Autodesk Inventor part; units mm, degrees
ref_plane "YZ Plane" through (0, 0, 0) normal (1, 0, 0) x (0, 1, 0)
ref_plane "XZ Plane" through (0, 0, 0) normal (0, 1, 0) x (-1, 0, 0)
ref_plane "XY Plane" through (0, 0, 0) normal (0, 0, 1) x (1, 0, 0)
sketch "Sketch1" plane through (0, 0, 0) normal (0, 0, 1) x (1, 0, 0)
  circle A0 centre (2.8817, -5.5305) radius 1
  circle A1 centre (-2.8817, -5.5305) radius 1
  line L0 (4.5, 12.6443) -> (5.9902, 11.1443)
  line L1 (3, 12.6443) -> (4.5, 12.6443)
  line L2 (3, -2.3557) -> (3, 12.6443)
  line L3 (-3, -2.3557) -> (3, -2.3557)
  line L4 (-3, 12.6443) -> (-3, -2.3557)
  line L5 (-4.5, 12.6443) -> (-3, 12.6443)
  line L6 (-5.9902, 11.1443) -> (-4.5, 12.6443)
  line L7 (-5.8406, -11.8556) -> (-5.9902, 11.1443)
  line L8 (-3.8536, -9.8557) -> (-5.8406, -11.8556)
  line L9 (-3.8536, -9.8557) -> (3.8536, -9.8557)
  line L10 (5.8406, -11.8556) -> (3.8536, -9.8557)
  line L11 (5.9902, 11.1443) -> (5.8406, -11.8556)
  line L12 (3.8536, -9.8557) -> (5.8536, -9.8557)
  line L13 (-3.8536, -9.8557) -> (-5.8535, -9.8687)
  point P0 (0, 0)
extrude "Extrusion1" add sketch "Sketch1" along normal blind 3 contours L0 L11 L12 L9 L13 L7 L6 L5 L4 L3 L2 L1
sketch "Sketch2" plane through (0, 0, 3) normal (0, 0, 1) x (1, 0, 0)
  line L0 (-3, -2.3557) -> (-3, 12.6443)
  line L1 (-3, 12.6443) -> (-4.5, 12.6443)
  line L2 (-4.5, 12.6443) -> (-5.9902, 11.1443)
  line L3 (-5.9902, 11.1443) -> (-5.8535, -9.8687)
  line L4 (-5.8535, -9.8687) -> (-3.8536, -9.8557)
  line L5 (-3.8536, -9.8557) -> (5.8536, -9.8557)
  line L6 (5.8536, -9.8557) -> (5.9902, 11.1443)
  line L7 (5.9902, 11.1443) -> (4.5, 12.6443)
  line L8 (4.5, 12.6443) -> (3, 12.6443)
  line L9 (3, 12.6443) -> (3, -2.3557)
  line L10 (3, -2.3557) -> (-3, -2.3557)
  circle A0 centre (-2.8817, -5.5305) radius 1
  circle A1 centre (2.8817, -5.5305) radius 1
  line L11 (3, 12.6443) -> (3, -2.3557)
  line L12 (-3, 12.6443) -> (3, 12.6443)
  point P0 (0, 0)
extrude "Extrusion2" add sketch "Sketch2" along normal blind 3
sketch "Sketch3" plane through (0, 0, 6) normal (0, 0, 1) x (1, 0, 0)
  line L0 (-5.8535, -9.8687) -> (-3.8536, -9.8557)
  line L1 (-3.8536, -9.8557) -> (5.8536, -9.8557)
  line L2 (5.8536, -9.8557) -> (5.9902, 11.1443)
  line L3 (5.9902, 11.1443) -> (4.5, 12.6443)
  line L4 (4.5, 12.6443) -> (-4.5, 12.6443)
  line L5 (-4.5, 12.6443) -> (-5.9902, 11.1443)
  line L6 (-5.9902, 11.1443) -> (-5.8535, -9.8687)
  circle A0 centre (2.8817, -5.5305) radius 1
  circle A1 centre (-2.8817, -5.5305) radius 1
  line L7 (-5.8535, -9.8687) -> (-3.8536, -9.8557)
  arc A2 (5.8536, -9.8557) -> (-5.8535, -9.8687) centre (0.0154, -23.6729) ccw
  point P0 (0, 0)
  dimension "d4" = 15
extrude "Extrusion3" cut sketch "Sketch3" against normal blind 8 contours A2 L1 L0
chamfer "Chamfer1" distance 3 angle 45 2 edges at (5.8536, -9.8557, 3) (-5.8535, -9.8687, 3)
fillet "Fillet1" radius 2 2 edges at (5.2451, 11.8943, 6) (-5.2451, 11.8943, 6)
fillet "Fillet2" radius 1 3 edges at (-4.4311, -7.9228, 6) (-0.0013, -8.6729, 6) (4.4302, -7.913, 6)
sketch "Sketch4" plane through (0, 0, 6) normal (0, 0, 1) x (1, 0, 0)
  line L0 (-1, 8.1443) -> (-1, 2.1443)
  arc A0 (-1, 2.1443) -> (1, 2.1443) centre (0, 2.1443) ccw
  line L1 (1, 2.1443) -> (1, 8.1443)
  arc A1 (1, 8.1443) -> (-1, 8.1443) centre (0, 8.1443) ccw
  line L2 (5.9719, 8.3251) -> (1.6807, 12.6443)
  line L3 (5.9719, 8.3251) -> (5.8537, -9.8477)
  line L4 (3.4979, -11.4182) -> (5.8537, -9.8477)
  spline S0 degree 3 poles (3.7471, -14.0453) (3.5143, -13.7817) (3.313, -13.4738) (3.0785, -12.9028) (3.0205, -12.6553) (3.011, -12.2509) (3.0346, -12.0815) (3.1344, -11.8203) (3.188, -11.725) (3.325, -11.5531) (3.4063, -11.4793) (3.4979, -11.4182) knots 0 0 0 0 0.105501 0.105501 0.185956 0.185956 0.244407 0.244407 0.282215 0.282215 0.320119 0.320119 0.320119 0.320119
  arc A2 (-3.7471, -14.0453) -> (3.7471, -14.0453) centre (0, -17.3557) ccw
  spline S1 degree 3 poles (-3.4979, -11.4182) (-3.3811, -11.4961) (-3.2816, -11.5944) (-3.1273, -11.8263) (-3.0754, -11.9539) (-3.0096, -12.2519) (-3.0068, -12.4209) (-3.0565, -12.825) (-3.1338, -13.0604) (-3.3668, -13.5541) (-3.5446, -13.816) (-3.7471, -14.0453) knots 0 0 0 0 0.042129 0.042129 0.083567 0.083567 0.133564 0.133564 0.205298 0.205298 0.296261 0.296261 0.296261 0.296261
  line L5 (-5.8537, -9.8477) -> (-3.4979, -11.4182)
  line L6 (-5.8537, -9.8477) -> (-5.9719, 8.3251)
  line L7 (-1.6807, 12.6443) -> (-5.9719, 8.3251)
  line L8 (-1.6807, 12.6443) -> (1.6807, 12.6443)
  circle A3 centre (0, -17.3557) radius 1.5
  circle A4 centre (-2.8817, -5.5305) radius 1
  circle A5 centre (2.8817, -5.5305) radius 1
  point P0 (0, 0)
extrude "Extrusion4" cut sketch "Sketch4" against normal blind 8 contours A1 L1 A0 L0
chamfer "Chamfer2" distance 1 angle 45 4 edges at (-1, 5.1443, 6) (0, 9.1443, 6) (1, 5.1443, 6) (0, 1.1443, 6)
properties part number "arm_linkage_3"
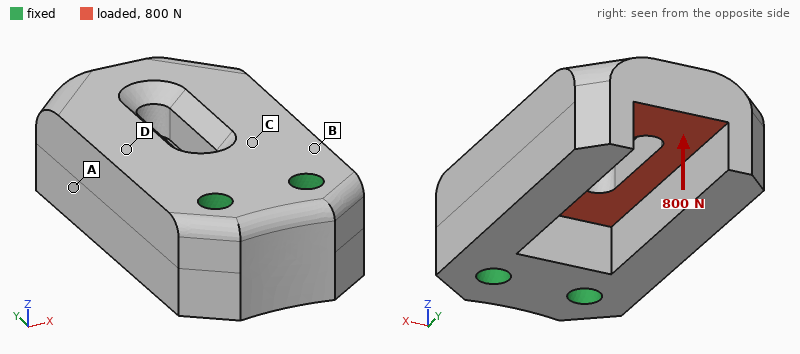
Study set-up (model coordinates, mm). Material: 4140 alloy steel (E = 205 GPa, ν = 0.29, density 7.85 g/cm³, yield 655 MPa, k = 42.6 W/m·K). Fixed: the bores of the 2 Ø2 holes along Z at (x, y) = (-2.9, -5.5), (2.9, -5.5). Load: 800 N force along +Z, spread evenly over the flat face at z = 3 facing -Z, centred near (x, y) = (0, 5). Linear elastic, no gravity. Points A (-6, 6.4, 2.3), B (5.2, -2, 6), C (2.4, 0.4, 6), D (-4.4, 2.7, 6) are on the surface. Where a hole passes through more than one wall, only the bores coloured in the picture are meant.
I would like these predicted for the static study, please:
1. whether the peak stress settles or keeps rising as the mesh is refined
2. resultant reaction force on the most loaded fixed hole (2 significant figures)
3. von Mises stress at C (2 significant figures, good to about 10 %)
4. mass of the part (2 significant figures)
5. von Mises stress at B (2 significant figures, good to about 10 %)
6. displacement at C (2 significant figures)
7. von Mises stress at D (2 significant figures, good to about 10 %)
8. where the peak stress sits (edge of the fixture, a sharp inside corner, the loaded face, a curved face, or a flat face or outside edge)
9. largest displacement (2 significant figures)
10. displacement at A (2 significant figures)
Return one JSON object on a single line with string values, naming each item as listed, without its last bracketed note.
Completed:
{"whether the peak stress settles or keeps rising as the mesh is refined": "keeps rising", "resultant reaction force on the most loaded fixed hole": "410 N", "von Mises stress at C": "87 MPa", "mass of the part": "8.7 g", "von Mises stress at B": "100 MPa", "displacement at C": "5.9 µm", "von Mises stress at D": "54 MPa", "where the peak stress sits": "edge of the fixture", "largest displacement": "28 µm", "displacement at A": "14 µm"}
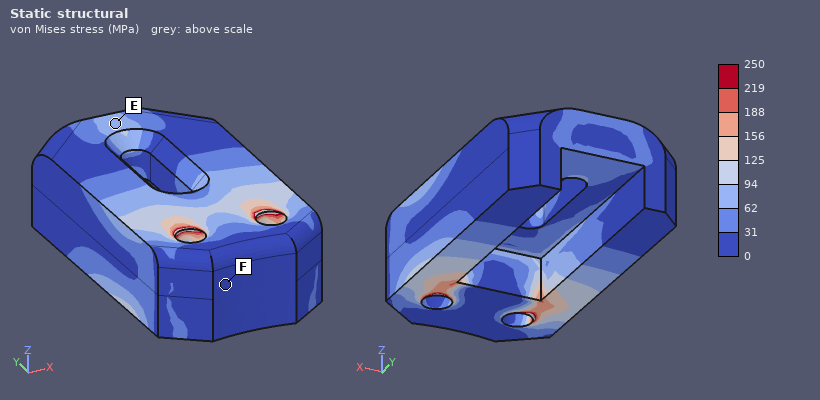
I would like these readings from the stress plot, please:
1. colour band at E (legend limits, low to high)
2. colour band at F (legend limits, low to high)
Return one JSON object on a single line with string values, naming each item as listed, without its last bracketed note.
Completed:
{"colour band at E": "62 to 94 MPa", "colour band at F": "0 to 31 MPa"}
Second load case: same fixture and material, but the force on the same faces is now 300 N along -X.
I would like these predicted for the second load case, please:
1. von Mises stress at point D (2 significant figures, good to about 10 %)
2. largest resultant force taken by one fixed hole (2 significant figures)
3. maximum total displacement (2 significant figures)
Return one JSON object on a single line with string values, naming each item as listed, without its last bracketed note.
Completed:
{"von Mises stress at point D": "11 MPa", "largest resultant force taken by one fixed hole": "440 N", "maximum total displacement": "6.6 µm"}
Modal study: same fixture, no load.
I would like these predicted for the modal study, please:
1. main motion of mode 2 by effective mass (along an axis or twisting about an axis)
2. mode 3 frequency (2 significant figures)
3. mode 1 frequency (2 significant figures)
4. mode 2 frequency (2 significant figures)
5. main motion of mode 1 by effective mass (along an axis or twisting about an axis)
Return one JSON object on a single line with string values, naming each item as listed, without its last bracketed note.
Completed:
{"main motion of mode 2 by effective mass": "along X", "mode 3 frequency": "27 kHz", "mode 1 frequency": "14 kHz", "mode 2 frequency": "18 kHz", "main motion of mode 1 by effective mass": "along Z"}
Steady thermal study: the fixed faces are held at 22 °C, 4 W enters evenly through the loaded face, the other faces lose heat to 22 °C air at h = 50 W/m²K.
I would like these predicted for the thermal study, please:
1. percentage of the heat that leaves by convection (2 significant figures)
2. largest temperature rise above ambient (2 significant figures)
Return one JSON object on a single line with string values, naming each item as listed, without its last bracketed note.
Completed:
{"percentage of the heat that leaves by convection": "9.5 %", "largest temperature rise above ambient": "20 K"}
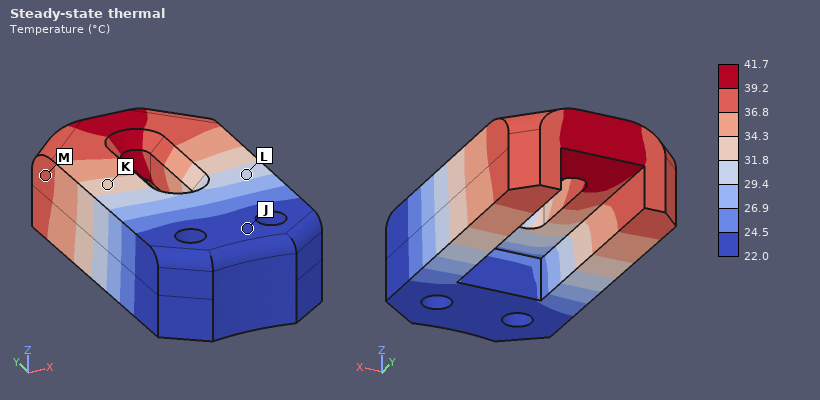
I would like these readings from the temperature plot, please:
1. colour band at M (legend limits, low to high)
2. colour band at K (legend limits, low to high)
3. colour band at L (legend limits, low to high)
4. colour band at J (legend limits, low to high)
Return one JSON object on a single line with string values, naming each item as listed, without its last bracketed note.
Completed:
{"colour band at M": "36.8 to 39.2 °C", "colour band at K": "31.8 to 34.3 °C", "colour band at L": "29.4 to 31.8 °C", "colour band at J": "22.0 to 24.5 °C"}
